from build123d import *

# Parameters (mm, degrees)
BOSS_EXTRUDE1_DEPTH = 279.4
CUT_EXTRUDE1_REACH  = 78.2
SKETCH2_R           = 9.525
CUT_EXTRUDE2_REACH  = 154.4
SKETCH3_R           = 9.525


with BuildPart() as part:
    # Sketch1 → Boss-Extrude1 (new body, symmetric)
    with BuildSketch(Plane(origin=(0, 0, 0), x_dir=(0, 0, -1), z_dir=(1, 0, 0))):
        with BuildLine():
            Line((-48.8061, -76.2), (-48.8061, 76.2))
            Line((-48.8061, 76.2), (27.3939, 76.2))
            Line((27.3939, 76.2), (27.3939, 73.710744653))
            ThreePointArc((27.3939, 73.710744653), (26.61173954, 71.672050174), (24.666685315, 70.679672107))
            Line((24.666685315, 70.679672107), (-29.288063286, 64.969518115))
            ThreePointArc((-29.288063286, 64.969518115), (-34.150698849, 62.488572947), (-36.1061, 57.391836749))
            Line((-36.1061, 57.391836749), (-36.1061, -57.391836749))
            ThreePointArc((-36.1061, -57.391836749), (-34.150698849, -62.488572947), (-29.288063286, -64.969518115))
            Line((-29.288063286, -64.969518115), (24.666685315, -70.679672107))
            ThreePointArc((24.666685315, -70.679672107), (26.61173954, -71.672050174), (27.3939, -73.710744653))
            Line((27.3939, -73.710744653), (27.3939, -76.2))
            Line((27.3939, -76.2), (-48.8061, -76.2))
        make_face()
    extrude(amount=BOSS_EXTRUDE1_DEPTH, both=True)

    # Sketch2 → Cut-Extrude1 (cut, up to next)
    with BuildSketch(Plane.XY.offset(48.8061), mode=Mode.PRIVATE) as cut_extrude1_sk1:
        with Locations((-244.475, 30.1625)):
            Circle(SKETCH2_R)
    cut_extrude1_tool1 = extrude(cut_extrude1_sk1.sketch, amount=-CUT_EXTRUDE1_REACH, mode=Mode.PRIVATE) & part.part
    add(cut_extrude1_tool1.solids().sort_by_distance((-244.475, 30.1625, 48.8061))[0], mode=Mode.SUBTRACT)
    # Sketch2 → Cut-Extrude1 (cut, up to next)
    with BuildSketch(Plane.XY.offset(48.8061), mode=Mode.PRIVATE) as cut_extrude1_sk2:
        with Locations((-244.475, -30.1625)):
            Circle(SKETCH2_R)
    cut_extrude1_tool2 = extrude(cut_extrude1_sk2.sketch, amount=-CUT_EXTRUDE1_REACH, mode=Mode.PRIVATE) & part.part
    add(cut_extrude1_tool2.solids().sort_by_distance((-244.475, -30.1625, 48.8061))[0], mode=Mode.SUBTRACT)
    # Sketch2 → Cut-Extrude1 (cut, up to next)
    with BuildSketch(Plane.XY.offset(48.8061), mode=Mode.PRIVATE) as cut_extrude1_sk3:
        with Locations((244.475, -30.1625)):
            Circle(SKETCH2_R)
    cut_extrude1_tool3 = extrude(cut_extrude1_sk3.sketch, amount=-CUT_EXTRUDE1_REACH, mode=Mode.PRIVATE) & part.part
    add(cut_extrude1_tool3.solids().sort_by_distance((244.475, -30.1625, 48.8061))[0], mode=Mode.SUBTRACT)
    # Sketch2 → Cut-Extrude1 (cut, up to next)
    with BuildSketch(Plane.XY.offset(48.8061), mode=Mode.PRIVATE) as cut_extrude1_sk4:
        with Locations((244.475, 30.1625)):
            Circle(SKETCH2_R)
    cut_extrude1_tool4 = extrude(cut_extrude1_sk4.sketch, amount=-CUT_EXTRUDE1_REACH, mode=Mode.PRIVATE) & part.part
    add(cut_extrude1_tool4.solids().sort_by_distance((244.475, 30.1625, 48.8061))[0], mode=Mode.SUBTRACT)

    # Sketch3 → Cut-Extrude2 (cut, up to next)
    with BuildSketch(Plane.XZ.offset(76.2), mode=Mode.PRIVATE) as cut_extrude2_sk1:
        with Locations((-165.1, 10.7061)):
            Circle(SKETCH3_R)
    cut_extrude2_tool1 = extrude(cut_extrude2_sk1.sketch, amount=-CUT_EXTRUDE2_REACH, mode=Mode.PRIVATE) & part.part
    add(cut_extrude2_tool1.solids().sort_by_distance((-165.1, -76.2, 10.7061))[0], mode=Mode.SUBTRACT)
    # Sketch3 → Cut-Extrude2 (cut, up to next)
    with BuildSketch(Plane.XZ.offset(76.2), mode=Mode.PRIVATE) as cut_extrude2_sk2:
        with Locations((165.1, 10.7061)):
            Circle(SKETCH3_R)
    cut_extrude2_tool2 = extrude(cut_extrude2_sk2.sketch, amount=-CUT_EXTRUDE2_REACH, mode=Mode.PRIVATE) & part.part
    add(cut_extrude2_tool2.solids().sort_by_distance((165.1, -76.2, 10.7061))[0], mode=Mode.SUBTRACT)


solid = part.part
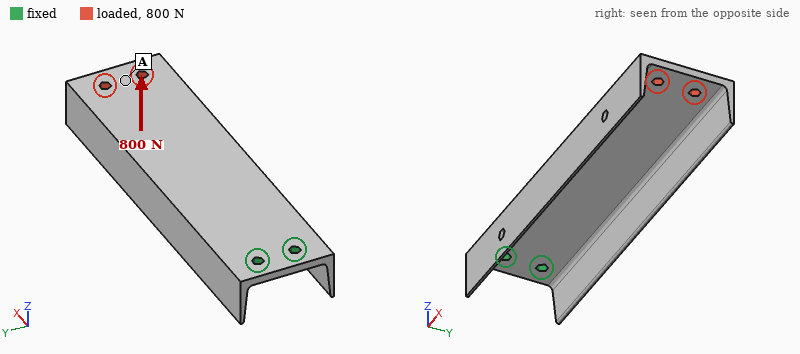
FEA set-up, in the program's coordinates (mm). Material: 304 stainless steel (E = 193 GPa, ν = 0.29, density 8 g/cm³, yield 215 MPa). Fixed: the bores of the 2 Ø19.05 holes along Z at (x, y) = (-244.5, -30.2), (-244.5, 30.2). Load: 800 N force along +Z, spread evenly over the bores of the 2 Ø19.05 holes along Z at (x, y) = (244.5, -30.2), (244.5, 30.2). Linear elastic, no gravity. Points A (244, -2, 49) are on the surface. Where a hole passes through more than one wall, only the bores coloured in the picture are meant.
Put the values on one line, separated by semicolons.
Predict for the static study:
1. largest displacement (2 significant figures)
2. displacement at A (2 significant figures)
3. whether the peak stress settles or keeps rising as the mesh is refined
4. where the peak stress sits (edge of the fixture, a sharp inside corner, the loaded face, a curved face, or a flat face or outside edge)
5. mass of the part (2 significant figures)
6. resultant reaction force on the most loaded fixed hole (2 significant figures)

0.72 mm; 0.66 mm; keeps rising; edge of the fixture; 13 kg; 650 N
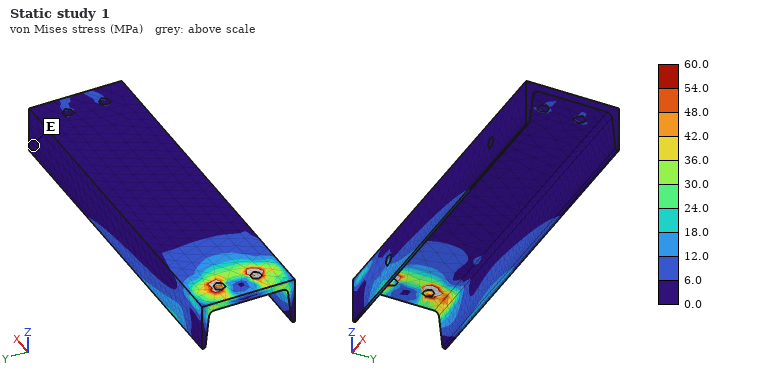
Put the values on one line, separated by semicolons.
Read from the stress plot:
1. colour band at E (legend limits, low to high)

0.0 to 6.0 MPa
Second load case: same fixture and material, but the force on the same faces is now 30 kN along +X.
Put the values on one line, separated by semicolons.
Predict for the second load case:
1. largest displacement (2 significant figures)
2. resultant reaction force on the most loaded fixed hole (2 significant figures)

0.19 mm; 15 kN
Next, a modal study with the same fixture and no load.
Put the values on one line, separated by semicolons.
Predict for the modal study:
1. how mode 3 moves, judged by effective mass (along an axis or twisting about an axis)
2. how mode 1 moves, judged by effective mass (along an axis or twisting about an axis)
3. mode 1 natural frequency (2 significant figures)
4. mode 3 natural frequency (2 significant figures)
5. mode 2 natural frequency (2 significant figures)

along Y; along Z; 82 Hz; 330 Hz; 190 Hz
